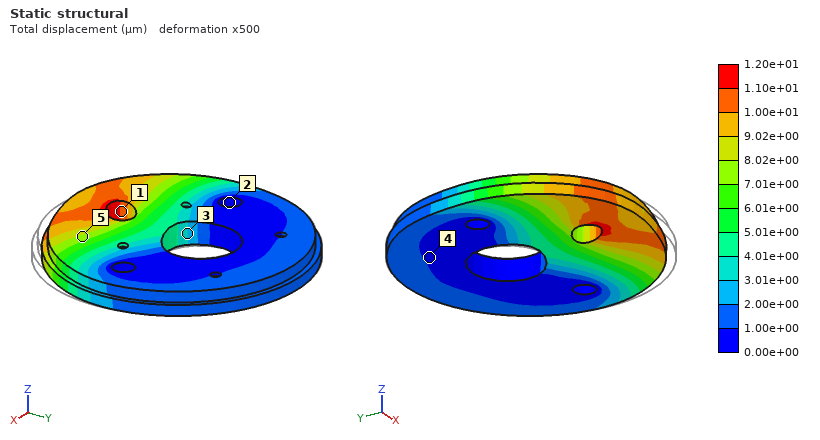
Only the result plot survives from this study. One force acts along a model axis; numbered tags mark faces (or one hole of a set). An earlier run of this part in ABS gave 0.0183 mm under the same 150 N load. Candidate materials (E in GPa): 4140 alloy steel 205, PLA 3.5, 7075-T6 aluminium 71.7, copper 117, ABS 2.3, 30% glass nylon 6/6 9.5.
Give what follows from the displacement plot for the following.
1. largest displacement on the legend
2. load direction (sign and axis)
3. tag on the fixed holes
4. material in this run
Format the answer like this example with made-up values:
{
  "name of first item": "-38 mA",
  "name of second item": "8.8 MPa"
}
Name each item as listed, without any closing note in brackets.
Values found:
{
  "largest displacement on the legend": "1.20e+01 µm",
  "load direction": "-X",
  "tag on the fixed holes": "2",
  "material in this run": "PLA"
}
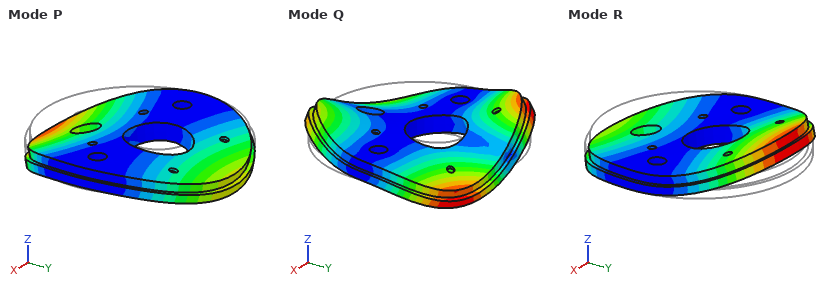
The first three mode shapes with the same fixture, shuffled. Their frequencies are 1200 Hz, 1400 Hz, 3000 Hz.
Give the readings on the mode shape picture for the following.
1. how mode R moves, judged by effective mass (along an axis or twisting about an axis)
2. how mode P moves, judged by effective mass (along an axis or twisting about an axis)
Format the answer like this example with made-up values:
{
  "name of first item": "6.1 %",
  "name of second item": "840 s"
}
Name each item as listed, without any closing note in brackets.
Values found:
{
  "how mode R moves, judged by effective mass": "twisting about X",
  "how mode P moves, judged by effective mass": "along Z"
}
